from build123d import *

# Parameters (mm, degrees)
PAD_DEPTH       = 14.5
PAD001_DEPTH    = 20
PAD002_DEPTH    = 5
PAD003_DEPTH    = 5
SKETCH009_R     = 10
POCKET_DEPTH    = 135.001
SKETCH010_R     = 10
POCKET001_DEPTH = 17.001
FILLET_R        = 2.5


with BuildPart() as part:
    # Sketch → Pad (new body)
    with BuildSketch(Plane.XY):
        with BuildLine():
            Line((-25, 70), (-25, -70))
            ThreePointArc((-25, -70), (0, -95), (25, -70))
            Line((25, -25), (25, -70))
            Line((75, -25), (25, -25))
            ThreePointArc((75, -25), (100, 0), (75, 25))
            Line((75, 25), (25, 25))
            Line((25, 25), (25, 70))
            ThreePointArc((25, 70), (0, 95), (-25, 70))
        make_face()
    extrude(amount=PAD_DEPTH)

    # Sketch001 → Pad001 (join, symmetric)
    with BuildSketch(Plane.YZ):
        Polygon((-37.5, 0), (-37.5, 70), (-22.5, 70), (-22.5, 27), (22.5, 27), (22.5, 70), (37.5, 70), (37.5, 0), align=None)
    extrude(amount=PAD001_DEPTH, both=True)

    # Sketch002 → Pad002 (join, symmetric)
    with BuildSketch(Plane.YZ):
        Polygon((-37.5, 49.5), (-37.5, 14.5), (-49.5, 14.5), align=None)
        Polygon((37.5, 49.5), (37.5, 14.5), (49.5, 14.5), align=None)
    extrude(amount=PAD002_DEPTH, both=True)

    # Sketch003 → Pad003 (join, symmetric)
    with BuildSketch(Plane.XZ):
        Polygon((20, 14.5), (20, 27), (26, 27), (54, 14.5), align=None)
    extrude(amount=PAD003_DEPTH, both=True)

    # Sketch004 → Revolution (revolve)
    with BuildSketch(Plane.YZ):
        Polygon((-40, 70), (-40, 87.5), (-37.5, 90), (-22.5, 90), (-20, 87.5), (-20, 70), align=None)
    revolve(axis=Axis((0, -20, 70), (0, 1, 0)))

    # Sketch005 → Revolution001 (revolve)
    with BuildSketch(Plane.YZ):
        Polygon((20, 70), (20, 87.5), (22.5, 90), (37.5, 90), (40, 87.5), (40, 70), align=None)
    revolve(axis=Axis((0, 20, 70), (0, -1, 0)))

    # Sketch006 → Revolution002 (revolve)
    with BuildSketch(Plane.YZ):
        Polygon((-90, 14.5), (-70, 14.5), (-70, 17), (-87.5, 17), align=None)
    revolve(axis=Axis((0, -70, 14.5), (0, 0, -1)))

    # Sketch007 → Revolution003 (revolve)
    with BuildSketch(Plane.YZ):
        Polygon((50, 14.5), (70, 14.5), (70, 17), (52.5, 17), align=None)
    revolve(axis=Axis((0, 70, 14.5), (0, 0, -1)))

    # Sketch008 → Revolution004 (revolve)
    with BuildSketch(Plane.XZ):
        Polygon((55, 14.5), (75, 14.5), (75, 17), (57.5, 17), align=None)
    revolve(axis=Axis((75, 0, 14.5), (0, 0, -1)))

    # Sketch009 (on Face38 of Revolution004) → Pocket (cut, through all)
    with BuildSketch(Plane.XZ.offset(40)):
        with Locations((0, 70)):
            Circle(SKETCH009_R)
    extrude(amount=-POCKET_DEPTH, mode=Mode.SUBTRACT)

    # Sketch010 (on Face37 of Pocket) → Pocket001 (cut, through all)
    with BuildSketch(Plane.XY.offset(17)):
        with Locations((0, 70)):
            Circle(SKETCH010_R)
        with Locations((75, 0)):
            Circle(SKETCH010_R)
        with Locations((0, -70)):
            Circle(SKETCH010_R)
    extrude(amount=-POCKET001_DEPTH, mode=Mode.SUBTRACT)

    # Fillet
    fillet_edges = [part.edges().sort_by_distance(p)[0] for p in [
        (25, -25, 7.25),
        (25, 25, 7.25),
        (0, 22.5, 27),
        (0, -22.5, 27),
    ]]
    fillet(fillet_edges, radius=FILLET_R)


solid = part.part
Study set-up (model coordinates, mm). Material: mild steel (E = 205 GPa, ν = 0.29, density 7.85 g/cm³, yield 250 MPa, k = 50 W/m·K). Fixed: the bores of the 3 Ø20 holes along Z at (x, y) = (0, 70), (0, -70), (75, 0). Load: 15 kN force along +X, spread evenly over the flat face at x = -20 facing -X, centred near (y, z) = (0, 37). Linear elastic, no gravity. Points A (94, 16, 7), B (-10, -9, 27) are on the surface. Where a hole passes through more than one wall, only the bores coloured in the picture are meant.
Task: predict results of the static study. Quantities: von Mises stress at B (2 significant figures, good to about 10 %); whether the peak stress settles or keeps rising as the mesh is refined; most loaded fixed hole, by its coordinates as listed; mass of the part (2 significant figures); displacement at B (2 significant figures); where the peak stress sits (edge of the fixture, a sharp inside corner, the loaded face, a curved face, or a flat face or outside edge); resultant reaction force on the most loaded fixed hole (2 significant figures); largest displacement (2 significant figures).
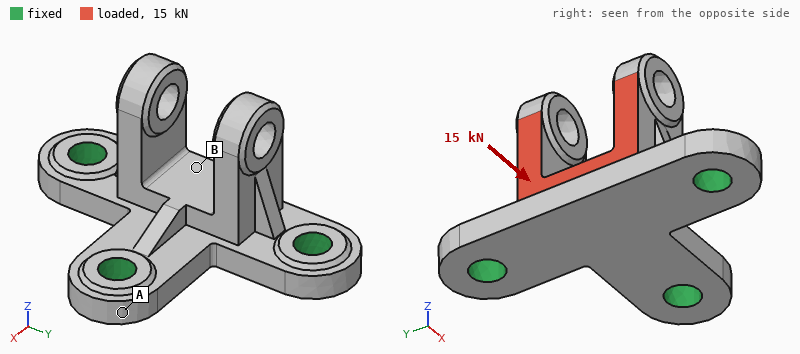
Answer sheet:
21 MPa
keeps rising
(75, 0)
2.2 kg
19 µm
edge of the fixture
10.0 kN
65 µm
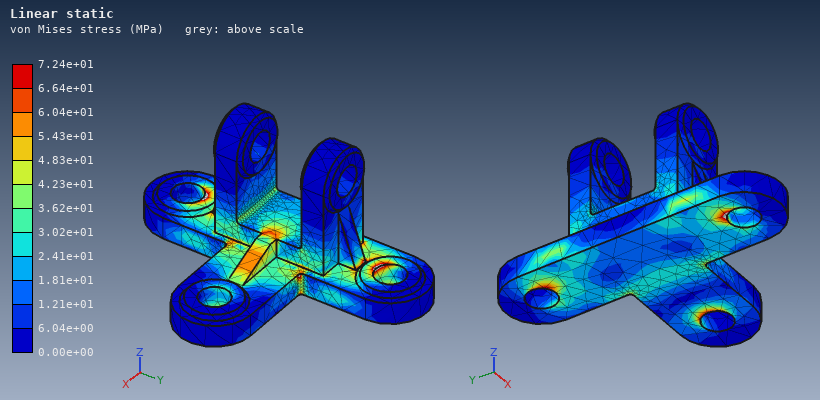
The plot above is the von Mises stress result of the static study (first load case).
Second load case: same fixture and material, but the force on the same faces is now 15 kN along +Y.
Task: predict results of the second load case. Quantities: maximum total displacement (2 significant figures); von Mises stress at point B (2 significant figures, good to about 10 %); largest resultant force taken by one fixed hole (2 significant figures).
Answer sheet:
51 µm
11 MPa
8.8 kN
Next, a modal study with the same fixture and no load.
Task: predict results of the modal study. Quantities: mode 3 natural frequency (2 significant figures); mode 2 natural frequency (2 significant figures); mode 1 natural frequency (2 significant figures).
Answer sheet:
3100 Hz
3100 Hz
2600 Hz
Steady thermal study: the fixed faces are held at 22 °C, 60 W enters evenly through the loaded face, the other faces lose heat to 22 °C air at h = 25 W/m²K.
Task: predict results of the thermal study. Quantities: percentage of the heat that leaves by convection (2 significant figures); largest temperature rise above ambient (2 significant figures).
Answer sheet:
26 %
34 K
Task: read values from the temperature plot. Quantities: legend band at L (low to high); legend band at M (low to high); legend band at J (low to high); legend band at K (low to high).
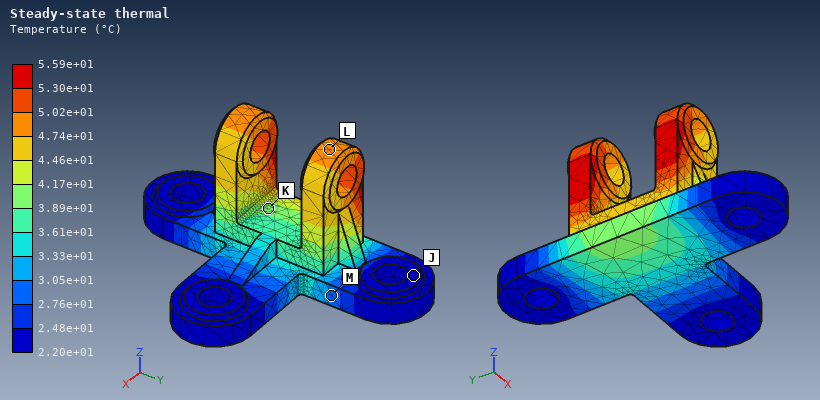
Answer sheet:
4.74e+01 to 5.02e+01 °C
2.76e+01 to 3.05e+01 °C
2.20e+01 to 2.48e+01 °C
3.89e+01 to 4.17e+01 °C
